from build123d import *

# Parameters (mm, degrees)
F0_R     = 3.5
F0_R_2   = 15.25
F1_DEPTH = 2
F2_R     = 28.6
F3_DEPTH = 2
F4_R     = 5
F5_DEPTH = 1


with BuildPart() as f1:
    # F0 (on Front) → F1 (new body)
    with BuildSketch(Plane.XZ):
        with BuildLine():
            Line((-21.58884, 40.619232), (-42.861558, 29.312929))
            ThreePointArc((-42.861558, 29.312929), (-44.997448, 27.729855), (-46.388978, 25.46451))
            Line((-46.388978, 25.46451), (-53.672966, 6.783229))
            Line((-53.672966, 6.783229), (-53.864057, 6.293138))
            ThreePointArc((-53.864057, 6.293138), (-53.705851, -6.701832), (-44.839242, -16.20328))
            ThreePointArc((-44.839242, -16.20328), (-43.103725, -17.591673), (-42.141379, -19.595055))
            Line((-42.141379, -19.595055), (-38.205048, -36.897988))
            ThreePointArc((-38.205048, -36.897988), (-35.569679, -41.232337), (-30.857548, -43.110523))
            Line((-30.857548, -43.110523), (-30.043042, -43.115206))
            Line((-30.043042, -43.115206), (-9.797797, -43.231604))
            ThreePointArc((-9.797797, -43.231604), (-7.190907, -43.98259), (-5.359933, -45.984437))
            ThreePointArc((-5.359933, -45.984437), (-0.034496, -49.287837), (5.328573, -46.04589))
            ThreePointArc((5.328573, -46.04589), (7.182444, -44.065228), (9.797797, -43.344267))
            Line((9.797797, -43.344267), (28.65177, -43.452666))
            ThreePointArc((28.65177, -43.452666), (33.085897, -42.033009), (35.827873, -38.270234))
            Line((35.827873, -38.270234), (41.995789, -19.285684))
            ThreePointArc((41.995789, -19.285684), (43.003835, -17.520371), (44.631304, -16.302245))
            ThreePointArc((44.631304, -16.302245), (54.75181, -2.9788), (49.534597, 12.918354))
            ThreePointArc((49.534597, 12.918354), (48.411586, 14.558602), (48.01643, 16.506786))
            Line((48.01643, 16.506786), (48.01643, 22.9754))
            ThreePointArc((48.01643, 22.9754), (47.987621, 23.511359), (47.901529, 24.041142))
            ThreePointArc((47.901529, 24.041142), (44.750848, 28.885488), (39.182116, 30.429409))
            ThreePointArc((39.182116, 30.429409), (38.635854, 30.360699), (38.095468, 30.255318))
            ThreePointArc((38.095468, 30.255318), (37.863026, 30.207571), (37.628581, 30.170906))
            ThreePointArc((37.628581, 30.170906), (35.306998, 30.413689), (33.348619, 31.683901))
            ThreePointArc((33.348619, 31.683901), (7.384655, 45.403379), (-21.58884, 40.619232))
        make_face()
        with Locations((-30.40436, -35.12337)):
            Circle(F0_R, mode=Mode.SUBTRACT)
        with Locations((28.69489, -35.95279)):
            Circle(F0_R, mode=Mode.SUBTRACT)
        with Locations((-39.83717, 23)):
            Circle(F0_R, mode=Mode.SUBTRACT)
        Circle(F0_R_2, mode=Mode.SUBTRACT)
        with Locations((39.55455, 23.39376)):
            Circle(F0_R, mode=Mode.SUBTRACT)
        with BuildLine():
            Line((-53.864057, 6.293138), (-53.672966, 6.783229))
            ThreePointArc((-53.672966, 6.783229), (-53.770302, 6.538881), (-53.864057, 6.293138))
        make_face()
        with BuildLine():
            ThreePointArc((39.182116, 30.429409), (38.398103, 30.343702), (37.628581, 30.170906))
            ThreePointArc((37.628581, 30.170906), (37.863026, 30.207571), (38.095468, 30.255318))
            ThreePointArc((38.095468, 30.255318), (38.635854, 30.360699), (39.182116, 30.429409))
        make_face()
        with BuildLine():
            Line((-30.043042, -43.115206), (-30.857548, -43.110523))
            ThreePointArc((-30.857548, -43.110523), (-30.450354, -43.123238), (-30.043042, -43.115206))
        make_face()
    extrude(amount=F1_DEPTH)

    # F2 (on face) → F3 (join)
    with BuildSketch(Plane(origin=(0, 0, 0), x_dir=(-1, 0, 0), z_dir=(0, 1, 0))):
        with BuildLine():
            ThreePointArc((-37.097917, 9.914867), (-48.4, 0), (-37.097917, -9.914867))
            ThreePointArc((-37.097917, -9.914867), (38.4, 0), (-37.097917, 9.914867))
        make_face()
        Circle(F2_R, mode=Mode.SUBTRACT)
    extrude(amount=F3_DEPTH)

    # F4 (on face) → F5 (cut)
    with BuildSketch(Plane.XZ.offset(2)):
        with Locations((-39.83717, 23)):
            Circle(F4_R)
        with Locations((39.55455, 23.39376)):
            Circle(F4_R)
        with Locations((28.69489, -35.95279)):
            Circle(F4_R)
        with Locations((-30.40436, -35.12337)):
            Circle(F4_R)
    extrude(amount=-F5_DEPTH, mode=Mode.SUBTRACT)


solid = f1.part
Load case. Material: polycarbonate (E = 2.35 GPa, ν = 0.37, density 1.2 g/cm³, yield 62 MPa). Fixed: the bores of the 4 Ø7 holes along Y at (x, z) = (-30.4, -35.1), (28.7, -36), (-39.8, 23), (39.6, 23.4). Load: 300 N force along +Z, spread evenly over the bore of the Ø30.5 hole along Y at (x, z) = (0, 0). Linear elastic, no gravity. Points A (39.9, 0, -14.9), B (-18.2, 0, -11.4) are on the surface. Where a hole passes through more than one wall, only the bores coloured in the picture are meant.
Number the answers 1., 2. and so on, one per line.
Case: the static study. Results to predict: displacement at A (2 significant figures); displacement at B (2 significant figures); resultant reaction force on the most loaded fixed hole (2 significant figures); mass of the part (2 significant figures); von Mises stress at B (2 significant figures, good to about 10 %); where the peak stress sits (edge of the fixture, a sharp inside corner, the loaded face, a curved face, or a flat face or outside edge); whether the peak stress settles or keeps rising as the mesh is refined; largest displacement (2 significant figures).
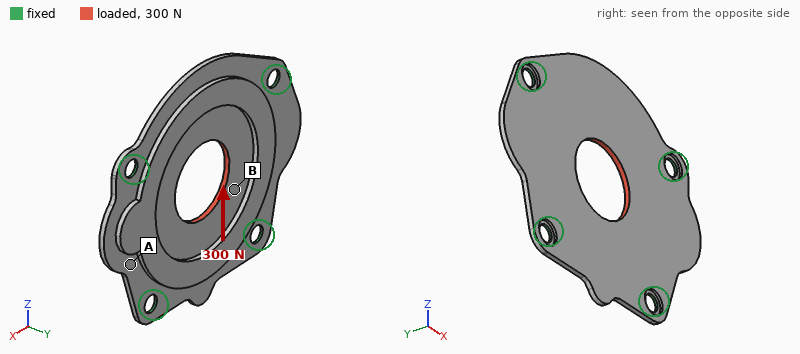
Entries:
1. 14 µm
2. 27 µm
3. 86 N
4. 21 g
5. 2.2 MPa
6. edge of the fixture
7. keeps rising
8. 80 µm
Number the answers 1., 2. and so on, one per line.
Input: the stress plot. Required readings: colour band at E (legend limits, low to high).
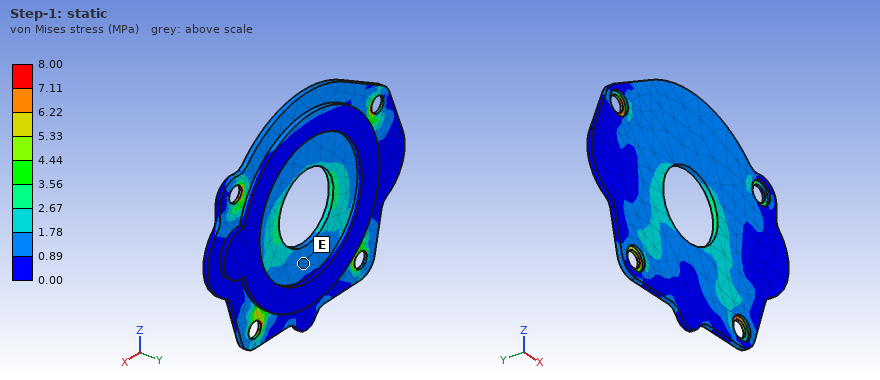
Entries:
1. 0.89 to 1.78 MPa
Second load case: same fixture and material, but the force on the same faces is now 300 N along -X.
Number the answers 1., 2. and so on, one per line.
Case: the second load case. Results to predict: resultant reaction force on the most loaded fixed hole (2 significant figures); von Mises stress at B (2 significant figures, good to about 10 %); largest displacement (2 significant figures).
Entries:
1. 86 N
2. 1.3 MPa
3. 44 µm
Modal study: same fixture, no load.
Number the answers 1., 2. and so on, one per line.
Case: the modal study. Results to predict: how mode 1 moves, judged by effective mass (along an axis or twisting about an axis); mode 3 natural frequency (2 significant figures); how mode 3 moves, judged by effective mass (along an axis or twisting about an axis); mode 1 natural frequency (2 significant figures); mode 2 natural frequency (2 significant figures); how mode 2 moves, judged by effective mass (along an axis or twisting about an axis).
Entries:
1. along Y
2. 880 Hz
3. twisting about Z
4. 490 Hz
5. 730 Hz
6. along Y
